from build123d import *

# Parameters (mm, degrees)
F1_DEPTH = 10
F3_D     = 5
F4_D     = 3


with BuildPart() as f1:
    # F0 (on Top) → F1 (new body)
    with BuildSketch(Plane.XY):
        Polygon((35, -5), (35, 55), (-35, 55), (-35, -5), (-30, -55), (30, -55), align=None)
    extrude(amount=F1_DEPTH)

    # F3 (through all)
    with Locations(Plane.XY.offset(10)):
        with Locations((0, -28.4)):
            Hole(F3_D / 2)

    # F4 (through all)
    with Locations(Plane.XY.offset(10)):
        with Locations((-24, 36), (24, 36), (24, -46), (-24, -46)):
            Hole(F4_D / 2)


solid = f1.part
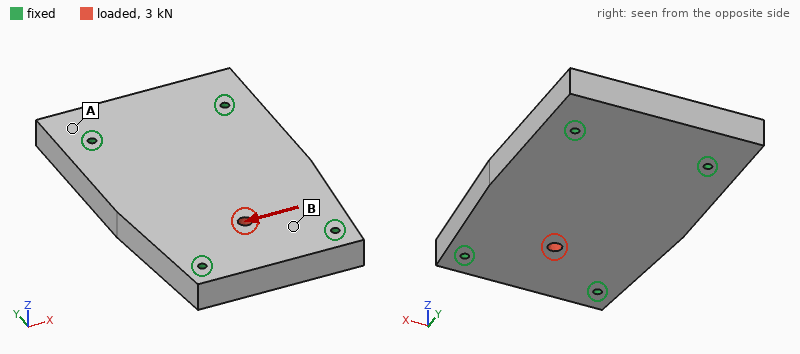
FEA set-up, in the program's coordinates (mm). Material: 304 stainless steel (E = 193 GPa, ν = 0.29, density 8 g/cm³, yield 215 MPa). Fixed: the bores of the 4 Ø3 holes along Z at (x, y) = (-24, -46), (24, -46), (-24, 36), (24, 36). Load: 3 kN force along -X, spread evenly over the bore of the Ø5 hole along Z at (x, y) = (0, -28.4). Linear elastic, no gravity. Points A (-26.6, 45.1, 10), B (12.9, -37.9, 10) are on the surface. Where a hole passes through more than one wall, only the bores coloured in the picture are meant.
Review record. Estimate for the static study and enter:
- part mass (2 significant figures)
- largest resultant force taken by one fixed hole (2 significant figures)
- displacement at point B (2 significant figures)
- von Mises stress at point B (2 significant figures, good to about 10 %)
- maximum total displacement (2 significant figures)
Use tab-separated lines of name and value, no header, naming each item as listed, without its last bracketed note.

part mass	590 g
largest resultant force taken by one fixed hole	1.2 kN
displacement at point B	0.78 µm
von Mises stress at point B	8.7 MPa
maximum total displacement	1.9 µm
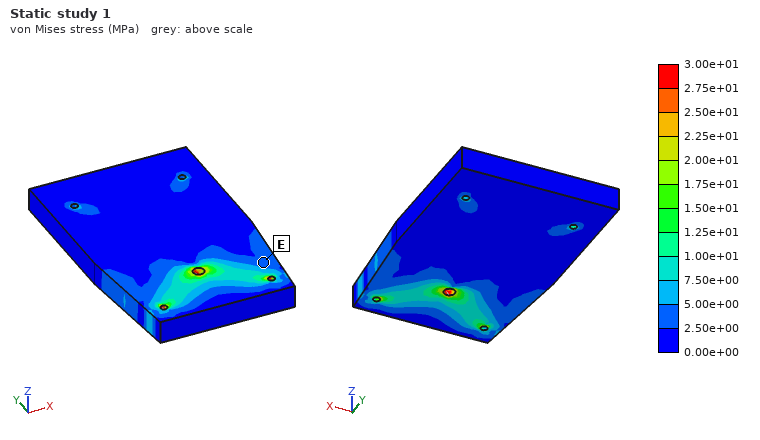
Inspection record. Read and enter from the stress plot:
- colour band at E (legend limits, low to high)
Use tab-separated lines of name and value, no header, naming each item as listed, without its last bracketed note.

colour band at E	2.50e+00 to 5.00e+00 MPa
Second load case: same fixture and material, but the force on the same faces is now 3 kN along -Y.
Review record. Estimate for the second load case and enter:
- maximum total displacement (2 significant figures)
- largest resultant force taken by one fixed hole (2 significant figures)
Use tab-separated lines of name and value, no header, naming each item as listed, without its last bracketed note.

maximum total displacement	1.7 µm
largest resultant force taken by one fixed hole	980 N
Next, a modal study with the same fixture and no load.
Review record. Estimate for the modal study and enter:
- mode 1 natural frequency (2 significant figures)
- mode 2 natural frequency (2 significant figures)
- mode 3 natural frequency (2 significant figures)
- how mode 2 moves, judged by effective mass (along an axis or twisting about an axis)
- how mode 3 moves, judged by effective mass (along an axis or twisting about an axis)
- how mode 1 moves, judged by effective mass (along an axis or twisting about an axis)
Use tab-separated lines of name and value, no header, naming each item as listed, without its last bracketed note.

mode 1 natural frequency	5300 Hz
mode 2 natural frequency	7600 Hz
mode 3 natural frequency	11 kHz
how mode 2 moves, judged by effective mass	twisting about Y
how mode 3 moves, judged by effective mass	along Z
how mode 1 moves, judged by effective mass	along Z
